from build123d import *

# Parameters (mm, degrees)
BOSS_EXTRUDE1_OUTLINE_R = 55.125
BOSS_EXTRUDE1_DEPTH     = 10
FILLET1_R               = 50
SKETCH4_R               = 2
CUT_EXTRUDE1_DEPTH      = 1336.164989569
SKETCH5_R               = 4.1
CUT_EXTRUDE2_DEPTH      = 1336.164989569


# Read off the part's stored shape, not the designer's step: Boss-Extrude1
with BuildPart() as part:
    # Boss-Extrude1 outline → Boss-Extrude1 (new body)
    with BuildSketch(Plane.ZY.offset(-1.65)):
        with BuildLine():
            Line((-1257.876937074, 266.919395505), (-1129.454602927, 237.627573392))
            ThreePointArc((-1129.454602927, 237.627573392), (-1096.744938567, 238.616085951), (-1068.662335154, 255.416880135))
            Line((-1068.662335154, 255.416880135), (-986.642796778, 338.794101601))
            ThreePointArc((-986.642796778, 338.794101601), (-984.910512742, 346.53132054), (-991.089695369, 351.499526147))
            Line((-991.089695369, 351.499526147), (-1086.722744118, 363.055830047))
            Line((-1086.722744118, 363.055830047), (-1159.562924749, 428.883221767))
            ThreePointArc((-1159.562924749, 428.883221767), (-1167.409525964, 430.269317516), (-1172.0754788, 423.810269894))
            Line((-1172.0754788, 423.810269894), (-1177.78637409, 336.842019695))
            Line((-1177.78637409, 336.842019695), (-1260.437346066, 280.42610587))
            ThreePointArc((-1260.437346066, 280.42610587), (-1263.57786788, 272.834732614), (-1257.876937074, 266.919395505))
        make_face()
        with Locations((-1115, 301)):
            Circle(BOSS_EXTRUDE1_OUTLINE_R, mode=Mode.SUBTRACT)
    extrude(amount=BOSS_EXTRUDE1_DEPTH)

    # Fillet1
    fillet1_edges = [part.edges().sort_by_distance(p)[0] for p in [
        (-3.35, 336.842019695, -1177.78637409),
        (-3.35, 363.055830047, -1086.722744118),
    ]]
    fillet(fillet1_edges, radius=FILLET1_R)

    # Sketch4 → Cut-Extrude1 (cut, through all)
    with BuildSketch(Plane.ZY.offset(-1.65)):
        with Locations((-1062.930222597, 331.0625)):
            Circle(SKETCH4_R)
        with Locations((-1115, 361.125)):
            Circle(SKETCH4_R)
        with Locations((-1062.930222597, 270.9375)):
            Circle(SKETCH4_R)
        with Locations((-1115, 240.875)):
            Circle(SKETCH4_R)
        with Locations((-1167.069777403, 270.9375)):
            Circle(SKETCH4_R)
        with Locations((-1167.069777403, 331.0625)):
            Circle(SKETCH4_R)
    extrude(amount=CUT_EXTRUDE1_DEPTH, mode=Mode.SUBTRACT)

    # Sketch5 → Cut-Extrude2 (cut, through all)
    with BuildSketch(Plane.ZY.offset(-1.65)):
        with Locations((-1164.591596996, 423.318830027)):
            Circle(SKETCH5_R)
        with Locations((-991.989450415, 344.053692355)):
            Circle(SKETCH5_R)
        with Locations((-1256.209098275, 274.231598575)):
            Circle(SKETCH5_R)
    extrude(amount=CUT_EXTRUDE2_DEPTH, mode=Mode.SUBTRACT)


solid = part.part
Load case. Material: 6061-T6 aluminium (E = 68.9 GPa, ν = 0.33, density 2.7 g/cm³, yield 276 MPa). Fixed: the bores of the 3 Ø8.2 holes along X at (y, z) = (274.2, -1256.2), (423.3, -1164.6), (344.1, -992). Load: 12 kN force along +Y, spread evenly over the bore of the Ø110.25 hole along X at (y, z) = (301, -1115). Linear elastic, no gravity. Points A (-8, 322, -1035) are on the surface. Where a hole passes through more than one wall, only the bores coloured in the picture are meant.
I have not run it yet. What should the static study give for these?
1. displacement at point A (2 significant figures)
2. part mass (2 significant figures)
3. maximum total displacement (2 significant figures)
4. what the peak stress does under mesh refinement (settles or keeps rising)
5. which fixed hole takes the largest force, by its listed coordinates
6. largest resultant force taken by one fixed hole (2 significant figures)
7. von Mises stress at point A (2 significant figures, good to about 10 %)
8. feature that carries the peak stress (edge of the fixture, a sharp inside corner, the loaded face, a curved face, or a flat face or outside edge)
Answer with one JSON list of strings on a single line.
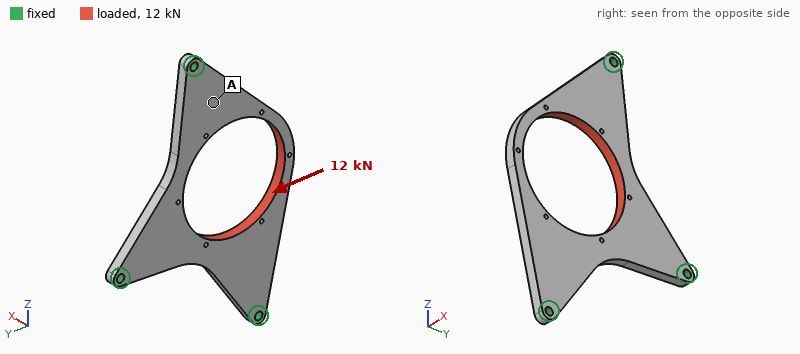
["50 µm", "430 g", "87 µm", "keeps rising", "(423.3, -1164.6)", "8.2 kN", "8.7 MPa", "edge of the fixture"]
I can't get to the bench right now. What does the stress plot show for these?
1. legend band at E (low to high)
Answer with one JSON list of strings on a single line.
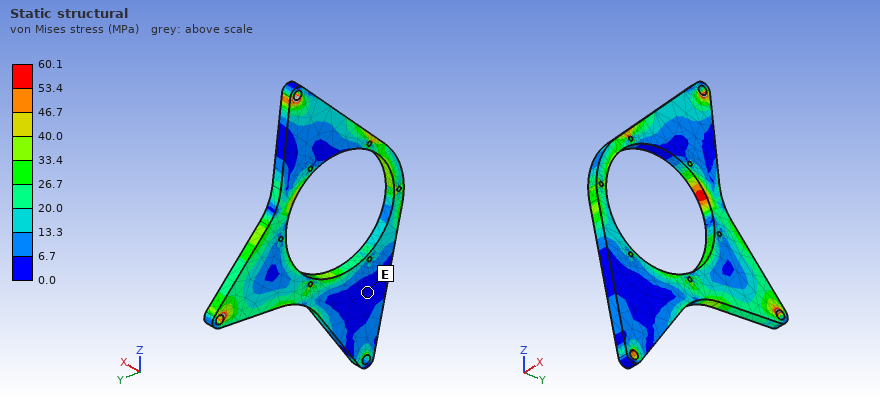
["0.0 to 6.7 MPa"]
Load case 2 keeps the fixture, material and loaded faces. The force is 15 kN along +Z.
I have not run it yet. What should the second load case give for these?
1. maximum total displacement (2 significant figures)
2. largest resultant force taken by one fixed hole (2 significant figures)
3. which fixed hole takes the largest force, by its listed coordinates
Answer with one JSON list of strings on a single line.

["0.12 mm", "7.8 kN", "(274.2, -1256.2)"]
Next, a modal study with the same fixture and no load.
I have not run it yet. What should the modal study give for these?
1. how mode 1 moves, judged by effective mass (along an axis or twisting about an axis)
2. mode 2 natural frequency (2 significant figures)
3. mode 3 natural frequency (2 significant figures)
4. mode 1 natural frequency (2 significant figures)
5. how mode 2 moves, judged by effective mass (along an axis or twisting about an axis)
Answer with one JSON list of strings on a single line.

["along X", "1300 Hz", "1400 Hz", "630 Hz", "along X"]
